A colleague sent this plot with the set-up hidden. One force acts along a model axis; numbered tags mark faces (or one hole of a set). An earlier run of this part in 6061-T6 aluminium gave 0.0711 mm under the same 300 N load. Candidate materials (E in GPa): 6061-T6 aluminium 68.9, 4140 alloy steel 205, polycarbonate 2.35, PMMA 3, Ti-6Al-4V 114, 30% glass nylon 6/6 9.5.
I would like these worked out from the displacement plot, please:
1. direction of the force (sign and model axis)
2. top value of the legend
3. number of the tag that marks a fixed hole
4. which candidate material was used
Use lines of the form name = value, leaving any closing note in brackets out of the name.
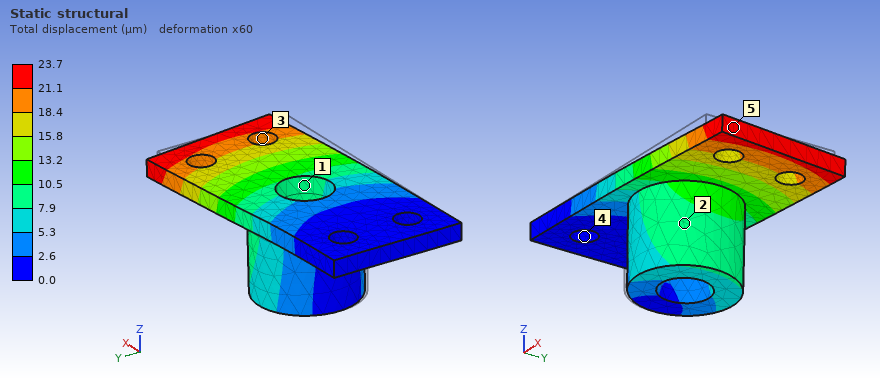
direction of the force = +Y
top value of the legend = 23.7 µm
number of the tag that marks a fixed hole = 4
which candidate material was used = 4140 alloy steel
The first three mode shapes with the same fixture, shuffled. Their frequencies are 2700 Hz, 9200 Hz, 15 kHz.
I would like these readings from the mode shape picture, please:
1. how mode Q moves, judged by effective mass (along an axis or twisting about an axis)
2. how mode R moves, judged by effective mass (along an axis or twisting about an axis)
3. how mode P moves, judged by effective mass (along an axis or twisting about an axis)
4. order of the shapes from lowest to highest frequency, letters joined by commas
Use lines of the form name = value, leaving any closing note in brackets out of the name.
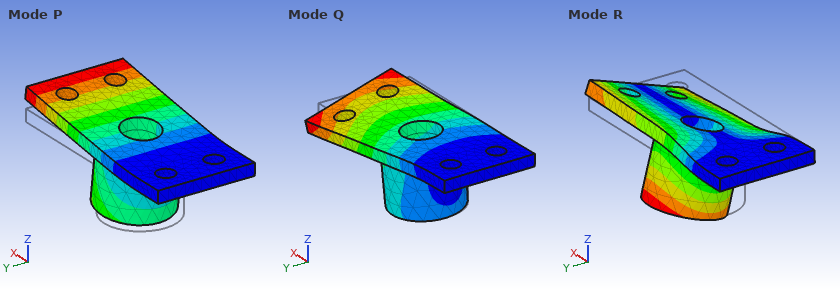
how mode Q moves, judged by effective mass = along Y
how mode R moves, judged by effective mass = along Y
how mode P moves, judged by effective mass = along Z
order of the shapes from lowest to highest frequency, letters joined by commas = P, R, Q
